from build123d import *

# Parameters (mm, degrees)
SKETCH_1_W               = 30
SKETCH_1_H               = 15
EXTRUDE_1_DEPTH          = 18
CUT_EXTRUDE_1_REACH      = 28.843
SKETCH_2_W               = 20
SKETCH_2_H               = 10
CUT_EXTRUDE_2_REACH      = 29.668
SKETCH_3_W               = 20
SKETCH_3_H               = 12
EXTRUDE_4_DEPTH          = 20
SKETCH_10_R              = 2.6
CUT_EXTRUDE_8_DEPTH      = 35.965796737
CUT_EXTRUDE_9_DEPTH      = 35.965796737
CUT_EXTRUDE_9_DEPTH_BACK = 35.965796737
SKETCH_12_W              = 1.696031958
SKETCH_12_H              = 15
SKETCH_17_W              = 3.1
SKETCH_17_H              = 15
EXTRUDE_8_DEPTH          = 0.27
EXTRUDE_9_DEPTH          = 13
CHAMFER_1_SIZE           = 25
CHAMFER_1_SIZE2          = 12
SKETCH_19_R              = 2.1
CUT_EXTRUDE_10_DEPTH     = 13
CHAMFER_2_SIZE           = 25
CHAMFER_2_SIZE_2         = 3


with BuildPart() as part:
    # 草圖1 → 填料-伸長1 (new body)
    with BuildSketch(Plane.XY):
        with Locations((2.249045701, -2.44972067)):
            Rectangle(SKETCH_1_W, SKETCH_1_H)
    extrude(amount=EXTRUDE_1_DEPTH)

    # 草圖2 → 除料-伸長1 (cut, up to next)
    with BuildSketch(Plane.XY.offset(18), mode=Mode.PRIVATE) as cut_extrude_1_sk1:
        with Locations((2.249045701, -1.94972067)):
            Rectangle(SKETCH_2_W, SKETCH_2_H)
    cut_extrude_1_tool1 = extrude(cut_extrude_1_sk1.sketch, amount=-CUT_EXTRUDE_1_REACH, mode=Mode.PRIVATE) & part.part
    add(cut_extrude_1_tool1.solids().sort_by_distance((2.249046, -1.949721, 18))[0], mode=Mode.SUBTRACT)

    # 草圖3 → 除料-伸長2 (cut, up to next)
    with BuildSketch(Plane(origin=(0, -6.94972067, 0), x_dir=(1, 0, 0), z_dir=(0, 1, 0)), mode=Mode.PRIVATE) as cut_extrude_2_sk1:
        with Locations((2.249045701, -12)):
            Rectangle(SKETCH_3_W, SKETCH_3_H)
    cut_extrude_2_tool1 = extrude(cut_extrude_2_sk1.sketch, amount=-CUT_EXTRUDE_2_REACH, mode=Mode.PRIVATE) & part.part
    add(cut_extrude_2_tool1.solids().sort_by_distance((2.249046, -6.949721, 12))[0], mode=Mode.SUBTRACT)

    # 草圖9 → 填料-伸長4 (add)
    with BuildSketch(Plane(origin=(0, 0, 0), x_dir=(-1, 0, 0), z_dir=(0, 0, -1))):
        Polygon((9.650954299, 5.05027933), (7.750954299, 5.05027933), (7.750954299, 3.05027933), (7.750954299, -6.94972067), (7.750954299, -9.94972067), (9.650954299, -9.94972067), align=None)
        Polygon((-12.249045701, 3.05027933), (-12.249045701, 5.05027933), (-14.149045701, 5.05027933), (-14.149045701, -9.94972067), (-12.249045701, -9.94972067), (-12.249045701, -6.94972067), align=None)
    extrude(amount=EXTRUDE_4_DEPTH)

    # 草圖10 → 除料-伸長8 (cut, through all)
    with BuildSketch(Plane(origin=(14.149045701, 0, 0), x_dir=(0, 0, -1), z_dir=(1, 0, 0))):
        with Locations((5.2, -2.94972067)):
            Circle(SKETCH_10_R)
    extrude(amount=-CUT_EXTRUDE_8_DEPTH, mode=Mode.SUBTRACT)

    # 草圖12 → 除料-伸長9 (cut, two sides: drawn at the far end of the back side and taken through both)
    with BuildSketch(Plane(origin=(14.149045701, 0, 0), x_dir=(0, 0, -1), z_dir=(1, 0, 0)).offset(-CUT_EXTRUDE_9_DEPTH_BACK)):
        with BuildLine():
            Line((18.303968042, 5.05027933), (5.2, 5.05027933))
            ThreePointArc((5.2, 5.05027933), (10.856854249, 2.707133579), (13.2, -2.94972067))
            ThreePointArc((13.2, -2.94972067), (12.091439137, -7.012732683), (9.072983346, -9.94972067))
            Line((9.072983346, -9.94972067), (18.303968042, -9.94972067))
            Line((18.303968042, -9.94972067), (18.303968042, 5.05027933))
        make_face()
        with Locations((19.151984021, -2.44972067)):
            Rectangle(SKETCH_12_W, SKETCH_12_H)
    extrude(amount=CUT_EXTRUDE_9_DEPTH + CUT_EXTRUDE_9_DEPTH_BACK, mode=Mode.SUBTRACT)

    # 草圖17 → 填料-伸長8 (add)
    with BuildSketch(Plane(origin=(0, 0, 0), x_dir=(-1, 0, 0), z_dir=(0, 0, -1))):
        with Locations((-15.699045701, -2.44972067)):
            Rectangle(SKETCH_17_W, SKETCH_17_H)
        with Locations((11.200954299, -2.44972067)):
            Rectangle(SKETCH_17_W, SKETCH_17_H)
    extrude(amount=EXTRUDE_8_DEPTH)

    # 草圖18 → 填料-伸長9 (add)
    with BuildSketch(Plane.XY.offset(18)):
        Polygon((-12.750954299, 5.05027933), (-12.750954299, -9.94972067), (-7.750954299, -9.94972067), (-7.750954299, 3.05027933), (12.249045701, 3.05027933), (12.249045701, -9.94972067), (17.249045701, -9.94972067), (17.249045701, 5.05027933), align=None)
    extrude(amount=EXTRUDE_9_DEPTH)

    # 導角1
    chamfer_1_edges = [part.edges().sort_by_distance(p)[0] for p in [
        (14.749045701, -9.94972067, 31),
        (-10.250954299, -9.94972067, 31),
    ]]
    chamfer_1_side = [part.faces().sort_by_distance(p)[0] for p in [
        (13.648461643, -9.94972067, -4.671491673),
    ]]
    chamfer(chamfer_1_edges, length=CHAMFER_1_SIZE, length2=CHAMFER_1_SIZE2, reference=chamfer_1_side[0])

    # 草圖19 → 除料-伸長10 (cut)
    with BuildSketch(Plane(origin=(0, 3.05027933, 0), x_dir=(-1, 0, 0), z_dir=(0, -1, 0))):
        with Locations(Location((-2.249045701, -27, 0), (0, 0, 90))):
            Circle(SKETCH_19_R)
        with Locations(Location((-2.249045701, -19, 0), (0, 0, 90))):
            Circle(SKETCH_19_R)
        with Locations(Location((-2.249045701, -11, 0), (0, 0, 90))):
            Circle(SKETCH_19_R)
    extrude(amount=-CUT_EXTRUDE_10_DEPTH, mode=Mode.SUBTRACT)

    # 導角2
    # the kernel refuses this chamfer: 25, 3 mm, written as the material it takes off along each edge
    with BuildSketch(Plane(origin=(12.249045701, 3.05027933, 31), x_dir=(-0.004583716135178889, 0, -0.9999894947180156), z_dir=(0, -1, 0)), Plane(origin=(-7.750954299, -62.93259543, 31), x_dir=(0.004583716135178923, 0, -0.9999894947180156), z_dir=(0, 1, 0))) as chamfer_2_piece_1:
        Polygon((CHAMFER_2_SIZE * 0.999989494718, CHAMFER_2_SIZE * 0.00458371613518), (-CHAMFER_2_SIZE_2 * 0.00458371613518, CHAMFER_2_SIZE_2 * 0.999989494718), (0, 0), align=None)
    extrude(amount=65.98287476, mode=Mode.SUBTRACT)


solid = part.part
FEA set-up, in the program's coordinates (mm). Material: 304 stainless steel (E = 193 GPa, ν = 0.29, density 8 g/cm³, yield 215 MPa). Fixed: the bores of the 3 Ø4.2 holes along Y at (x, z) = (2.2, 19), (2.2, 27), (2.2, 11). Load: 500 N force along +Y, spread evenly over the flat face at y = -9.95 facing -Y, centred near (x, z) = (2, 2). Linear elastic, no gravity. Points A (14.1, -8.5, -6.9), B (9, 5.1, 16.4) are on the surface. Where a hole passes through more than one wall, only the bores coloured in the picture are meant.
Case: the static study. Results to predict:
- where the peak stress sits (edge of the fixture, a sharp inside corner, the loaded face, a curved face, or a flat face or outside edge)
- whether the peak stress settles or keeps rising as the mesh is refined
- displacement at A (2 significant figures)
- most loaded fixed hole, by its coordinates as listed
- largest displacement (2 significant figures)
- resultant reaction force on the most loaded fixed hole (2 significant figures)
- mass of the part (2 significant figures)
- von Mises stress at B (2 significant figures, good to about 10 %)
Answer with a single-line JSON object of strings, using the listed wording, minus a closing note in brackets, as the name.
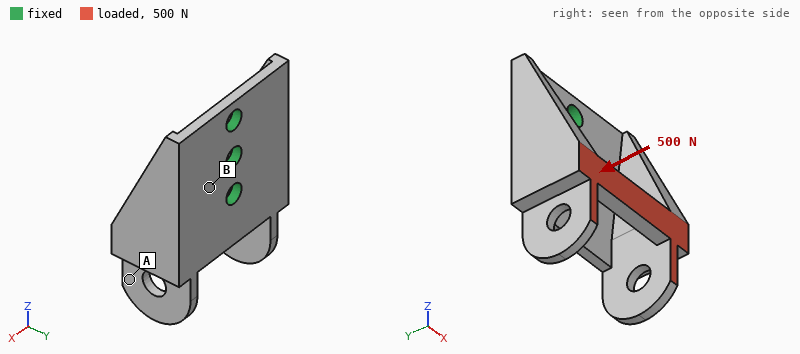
{"where the peak stress sits": "edge of the fixture", "whether the peak stress settles or keeps rising as the mesh is refined": "keeps rising", "displacement at A": "50 µm", "most loaded fixed hole, by its coordinates as listed": "(2.2, 11)", "largest displacement": "58 µm", "resultant reaction force on the most loaded fixed hole": "660 N", "mass of the part": "39 g", "von Mises stress at B": "53 MPa"}
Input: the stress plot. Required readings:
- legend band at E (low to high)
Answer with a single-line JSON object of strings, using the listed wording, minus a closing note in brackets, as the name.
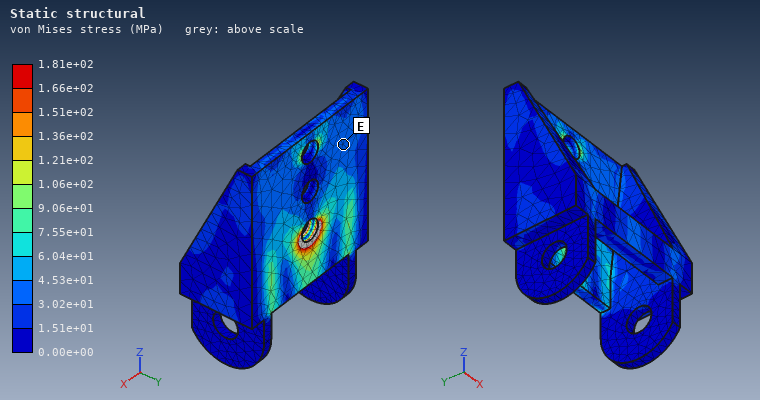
{"legend band at E": "3.02e+01 to 4.53e+01 MPa"}
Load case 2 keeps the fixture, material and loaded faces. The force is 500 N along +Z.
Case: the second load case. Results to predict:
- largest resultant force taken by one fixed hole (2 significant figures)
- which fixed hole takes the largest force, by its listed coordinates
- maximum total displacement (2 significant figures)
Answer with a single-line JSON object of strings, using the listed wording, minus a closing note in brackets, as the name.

{"largest resultant force taken by one fixed hole": "480 N", "which fixed hole takes the largest force, by its listed coordinates": "(2.2, 11)", "maximum total displacement": "59 µm"}
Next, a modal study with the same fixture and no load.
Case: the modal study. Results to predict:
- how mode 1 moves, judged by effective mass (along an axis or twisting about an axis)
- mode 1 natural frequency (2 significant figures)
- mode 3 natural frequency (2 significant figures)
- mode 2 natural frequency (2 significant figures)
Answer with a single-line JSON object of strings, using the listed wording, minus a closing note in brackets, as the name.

{"how mode 1 moves, judged by effective mass": "along X", "mode 1 natural frequency": "2600 Hz", "mode 3 natural frequency": "6500 Hz", "mode 2 natural frequency": "3800 Hz"}
